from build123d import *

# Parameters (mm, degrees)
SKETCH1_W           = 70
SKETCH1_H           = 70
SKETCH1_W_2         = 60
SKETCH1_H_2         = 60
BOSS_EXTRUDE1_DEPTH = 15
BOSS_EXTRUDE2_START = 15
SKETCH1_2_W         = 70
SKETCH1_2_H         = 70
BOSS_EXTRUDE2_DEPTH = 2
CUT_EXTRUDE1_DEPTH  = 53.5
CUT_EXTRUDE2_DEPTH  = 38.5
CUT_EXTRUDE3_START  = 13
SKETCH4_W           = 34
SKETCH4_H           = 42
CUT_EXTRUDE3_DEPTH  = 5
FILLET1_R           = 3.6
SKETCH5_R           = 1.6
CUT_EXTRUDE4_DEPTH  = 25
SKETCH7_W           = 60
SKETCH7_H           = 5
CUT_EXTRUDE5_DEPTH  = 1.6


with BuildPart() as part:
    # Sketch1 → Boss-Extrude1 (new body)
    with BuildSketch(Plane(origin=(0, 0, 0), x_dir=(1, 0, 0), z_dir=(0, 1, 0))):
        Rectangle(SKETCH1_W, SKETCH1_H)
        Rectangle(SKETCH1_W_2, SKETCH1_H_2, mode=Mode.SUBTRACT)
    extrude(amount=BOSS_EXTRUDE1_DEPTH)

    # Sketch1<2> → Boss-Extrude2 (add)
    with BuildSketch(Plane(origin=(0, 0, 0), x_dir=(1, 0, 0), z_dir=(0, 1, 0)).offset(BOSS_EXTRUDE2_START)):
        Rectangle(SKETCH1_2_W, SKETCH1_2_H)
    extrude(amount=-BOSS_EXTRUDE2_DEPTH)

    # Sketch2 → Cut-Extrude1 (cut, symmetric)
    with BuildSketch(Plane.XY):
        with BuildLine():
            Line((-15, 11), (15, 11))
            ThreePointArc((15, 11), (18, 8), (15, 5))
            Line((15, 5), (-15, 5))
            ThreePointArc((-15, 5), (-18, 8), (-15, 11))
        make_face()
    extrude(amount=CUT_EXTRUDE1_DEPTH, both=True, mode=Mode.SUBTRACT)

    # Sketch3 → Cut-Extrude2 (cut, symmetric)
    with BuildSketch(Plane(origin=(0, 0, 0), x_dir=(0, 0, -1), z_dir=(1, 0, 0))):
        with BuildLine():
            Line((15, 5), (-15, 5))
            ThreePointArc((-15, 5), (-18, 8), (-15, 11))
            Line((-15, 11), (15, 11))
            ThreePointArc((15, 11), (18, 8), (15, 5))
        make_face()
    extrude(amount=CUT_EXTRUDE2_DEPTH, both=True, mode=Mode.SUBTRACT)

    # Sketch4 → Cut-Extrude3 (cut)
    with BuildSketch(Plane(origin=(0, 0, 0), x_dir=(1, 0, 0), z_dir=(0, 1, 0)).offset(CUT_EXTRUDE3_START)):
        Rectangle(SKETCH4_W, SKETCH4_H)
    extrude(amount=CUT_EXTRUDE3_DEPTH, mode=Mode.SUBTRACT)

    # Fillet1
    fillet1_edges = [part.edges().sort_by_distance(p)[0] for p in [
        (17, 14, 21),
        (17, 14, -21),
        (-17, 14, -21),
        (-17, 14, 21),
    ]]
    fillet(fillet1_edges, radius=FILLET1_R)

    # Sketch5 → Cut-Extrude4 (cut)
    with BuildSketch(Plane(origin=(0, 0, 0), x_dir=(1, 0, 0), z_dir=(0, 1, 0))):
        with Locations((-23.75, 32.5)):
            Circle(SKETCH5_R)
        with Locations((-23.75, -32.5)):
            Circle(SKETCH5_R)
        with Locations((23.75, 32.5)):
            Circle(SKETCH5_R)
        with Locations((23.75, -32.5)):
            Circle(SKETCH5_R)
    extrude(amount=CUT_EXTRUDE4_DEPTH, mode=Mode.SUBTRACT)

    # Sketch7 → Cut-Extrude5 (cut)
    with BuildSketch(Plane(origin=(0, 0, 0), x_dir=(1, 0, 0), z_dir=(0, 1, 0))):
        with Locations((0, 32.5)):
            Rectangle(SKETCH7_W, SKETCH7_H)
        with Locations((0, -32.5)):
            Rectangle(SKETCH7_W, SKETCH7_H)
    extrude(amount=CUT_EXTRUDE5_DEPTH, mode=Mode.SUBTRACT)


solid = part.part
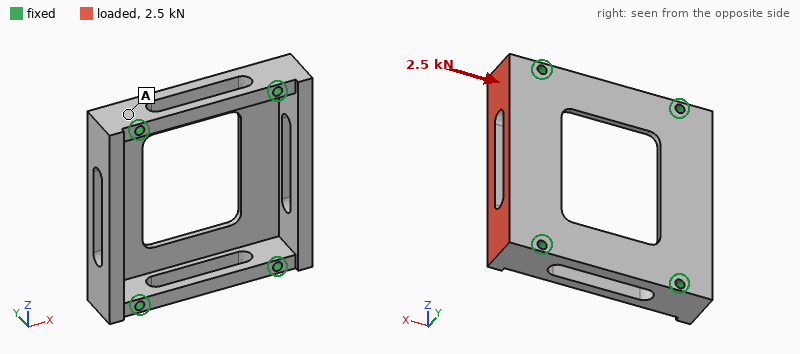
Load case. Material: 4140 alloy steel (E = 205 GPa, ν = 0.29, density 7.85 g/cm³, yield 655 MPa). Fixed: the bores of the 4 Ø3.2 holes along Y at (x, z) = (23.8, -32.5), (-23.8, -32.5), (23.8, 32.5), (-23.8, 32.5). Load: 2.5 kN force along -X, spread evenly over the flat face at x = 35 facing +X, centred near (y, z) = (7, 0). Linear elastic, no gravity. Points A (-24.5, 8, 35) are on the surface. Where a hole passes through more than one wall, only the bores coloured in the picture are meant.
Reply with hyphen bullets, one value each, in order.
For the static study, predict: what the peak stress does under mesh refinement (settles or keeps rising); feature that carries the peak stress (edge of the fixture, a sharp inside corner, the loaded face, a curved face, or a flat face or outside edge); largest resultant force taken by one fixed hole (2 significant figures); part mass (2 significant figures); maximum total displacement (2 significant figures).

- keeps rising
- a sharp inside corner
- 1.2 kN
- 140 g
- 44 µm
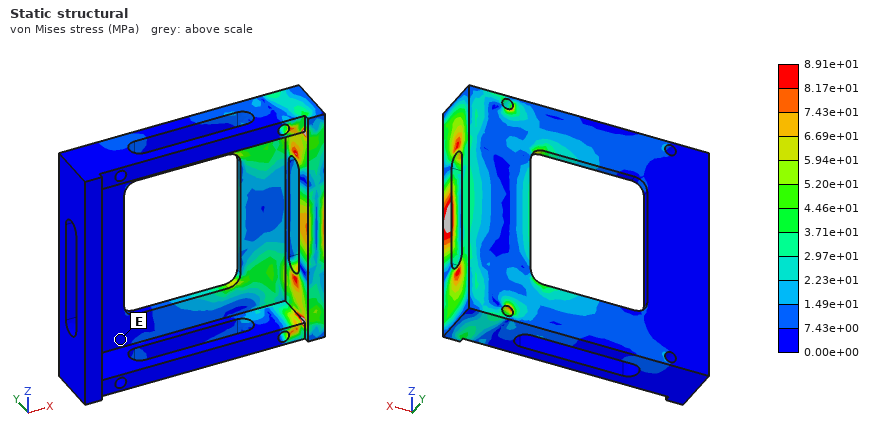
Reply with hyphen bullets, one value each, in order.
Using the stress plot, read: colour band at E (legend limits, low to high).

- 0.00e+00 to 7.43e+00 MPa
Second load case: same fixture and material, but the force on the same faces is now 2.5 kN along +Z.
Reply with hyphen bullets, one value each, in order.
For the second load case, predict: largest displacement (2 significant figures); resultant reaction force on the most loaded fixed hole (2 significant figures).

- 7.4 µm
- 1.3 kN
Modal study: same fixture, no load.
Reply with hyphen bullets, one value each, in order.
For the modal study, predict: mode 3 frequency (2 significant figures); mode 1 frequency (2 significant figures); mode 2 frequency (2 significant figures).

- 8100 Hz
- 6200 Hz
- 6400 Hz
